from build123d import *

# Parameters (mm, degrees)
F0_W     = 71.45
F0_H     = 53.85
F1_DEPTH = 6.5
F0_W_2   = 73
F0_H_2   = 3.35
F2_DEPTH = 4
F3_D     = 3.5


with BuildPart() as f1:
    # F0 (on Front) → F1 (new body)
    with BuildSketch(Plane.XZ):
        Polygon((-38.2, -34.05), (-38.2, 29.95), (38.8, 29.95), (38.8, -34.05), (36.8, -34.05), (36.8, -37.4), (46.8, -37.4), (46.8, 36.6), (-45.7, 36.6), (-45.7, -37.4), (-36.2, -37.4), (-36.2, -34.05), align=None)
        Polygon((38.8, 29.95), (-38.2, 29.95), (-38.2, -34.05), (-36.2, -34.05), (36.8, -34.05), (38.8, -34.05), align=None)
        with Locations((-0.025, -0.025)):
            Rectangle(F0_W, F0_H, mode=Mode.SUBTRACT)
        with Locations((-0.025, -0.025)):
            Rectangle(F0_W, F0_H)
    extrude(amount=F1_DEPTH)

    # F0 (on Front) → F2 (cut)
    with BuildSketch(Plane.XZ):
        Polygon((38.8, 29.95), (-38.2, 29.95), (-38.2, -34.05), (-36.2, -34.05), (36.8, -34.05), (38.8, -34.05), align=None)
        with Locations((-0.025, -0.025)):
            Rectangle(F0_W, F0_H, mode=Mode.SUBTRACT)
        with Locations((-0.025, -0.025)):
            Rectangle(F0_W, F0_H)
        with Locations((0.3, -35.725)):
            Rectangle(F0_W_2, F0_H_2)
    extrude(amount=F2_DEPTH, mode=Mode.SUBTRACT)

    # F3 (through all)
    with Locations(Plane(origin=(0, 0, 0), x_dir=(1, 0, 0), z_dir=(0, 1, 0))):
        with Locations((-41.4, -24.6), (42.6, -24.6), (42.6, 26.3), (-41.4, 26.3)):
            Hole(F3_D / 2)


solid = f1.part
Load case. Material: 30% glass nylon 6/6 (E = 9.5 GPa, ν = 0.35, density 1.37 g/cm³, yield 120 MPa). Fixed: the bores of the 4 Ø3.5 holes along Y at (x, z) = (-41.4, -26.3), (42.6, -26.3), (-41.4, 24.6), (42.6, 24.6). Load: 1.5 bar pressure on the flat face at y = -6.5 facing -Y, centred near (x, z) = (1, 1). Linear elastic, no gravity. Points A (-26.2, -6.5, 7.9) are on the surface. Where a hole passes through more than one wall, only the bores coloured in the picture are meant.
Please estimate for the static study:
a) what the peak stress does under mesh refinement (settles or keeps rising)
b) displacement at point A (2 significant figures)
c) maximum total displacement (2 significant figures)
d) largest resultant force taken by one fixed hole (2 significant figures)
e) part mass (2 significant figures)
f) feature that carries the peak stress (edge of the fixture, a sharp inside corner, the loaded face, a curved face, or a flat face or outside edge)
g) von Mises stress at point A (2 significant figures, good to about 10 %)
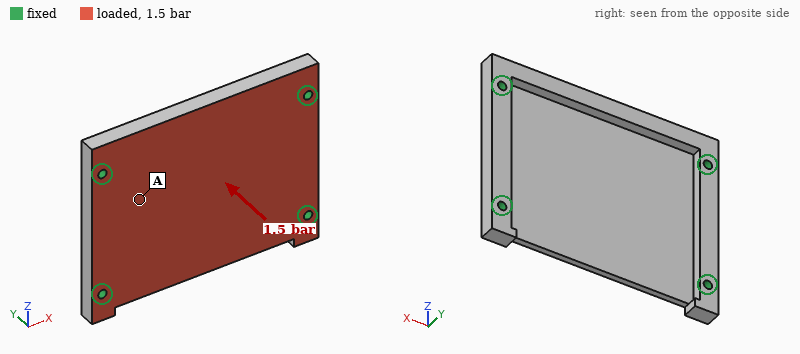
keeps rising
0.37 mm
1.4 mm
290 N
31 g
edge of the fixture
10 MPa
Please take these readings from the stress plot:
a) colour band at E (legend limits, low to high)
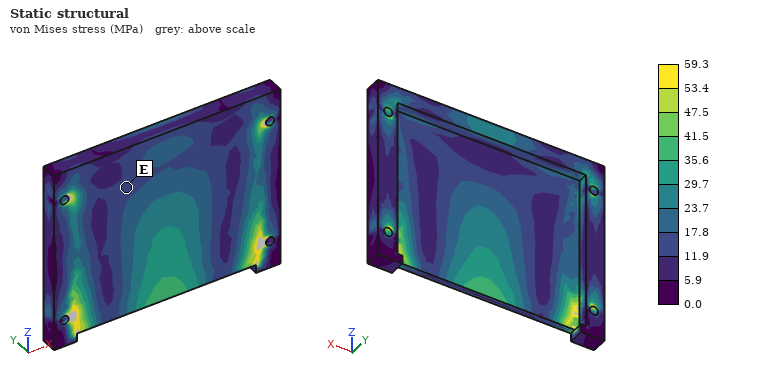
11.9 to 17.8 MPa
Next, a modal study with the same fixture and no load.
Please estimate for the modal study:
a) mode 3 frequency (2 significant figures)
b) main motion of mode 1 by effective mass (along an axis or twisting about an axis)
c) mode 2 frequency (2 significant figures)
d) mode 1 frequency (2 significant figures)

2500 Hz
along Y
1800 Hz
1200 Hz
